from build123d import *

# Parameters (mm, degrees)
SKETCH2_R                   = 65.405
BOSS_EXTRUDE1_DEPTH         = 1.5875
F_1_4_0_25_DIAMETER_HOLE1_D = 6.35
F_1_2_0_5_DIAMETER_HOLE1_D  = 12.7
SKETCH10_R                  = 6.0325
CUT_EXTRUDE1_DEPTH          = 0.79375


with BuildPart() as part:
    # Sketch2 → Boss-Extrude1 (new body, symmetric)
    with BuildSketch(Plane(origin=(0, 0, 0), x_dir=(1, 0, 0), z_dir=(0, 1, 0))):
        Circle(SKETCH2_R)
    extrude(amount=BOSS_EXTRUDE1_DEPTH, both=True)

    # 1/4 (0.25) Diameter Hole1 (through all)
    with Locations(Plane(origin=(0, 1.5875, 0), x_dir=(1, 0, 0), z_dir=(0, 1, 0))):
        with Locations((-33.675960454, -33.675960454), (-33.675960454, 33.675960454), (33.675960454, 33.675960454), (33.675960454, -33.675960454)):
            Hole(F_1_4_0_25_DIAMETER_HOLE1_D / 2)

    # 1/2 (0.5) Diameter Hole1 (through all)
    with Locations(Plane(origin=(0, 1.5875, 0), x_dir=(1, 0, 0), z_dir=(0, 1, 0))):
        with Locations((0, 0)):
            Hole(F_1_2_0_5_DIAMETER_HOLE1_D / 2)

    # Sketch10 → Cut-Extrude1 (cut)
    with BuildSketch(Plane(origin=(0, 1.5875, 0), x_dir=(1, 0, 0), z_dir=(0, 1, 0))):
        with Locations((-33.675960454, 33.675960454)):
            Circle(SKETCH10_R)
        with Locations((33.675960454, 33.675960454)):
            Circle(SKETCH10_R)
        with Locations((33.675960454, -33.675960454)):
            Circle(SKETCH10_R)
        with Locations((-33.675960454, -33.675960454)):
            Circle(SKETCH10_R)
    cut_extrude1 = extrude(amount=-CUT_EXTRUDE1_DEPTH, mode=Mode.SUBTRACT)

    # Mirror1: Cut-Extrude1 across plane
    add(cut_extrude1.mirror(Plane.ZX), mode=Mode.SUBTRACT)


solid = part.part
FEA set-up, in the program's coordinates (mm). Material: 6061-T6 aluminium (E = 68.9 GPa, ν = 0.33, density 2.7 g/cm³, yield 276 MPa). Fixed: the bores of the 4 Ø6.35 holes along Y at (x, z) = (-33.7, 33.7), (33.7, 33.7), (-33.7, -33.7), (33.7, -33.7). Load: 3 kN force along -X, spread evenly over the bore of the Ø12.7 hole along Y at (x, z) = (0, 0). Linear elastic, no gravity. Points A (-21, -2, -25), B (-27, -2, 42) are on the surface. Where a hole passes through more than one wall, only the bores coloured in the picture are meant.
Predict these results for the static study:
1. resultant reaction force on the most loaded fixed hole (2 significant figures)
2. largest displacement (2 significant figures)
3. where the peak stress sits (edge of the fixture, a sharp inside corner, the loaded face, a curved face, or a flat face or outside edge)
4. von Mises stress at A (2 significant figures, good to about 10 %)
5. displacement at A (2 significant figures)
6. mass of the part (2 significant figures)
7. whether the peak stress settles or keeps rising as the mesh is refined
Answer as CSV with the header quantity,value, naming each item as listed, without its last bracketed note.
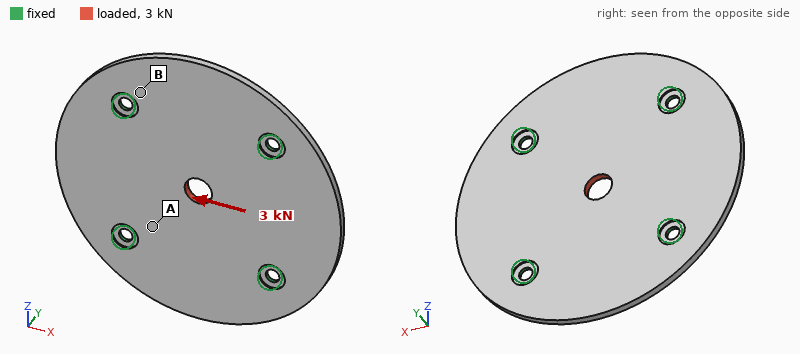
quantity,value
resultant reaction force on the most loaded fixed hole,770 N
largest displacement,10 µm
where the peak stress sits,edge of the fixture
von Mises stress at A,9.8 MPa
displacement at A,3.2 µm
mass of the part,110 g
whether the peak stress settles or keeps rising as the mesh is refined,keeps rising
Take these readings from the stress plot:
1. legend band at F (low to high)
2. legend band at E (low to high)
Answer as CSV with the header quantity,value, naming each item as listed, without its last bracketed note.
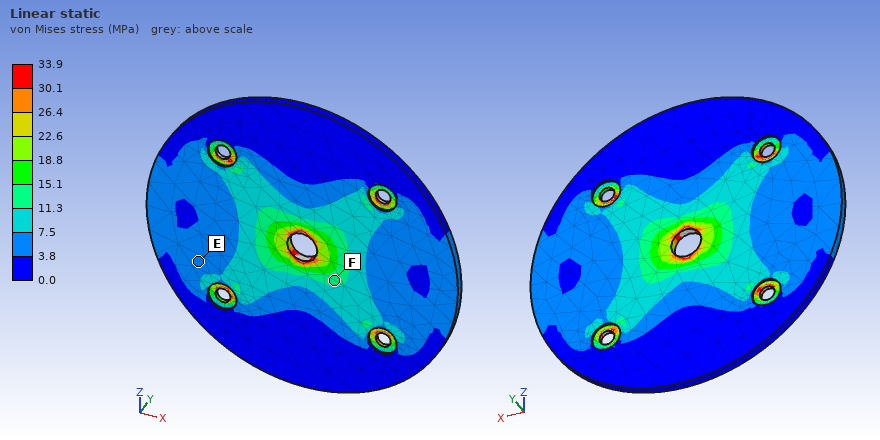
quantity,value
legend band at F,11.3 to 15.1 MPa
legend band at E,3.8 to 7.5 MPa
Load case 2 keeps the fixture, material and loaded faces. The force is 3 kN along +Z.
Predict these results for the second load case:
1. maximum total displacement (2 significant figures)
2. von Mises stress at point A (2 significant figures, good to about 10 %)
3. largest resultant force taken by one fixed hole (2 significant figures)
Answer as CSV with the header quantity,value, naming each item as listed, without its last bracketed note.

quantity,value
maximum total displacement,10 µm
von Mises stress at point A,9.8 MPa
largest resultant force taken by one fixed hole,770 N
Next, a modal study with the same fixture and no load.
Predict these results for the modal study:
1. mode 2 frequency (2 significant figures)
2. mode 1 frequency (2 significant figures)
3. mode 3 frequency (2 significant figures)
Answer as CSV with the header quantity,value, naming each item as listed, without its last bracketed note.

quantity,value
mode 2 frequency,1900 Hz
mode 1 frequency,1600 Hz
mode 3 frequency,1900 Hz
